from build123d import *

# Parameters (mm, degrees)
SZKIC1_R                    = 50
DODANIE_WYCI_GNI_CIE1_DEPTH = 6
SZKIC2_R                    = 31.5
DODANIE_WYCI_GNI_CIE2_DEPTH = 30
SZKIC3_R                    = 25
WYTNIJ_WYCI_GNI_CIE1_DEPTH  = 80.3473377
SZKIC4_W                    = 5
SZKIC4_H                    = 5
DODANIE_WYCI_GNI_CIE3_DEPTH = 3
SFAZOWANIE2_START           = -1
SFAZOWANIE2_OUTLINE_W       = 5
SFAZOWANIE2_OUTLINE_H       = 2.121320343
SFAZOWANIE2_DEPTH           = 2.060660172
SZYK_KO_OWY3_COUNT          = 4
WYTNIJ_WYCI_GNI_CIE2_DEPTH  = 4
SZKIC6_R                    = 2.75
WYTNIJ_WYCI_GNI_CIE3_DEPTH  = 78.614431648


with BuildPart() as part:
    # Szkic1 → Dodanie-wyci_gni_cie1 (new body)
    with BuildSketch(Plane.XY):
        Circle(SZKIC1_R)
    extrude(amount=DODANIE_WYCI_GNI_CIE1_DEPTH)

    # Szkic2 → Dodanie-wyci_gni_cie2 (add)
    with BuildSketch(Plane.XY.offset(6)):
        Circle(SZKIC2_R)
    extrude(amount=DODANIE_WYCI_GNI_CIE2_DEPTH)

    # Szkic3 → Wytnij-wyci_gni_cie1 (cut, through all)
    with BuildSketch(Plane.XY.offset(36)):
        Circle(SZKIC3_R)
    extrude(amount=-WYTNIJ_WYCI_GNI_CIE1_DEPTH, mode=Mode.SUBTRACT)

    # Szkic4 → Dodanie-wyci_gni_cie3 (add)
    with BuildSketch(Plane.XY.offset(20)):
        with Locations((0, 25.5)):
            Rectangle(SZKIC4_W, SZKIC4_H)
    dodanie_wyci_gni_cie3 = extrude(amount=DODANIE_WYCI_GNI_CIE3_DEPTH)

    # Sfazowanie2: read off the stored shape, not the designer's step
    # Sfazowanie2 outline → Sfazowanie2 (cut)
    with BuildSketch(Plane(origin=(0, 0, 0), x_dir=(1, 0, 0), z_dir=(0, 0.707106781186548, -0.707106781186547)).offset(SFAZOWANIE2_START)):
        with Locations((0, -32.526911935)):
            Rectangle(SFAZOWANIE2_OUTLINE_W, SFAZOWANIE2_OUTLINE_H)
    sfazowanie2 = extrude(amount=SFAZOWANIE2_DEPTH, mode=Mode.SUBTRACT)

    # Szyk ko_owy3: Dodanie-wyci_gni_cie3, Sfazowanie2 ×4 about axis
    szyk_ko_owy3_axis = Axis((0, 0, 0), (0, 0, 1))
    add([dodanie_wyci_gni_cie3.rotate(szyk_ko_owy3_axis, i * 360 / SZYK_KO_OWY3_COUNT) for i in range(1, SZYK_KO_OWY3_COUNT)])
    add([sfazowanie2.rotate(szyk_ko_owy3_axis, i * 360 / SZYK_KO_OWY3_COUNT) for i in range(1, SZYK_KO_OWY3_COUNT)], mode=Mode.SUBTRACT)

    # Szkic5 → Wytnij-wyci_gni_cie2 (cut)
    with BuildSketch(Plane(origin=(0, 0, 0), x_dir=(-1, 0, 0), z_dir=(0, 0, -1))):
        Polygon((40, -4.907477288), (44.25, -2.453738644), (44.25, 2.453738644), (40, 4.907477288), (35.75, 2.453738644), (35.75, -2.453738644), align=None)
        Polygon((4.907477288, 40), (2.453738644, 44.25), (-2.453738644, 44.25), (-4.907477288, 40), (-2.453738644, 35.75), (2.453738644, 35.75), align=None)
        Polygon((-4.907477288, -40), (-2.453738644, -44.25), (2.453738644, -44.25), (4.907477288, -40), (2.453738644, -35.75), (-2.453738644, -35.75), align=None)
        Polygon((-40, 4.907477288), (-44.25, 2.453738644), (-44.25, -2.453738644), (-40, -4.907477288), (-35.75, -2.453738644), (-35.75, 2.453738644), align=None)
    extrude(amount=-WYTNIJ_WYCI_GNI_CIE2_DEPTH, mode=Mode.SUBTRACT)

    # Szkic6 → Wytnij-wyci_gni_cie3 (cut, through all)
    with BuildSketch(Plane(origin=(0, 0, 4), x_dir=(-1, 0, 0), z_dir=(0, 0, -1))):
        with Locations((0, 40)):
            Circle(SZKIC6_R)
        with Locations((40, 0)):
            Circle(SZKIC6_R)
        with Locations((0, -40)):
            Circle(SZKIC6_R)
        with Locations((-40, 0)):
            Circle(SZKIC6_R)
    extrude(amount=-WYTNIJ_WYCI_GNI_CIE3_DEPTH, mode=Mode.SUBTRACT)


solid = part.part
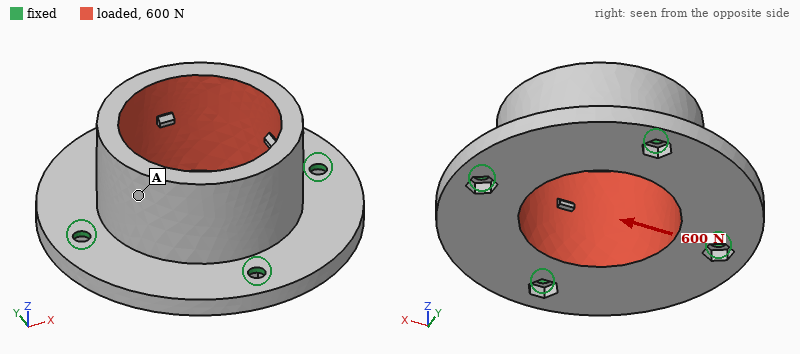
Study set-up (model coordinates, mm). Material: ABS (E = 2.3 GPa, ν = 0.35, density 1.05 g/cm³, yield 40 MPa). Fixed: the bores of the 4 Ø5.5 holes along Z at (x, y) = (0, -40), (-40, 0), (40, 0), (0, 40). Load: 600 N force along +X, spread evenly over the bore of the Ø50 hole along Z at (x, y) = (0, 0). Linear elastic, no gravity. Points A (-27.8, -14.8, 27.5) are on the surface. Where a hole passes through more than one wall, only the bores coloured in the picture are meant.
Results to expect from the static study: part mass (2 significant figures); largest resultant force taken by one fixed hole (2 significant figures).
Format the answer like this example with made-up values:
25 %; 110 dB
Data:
72 g; 180 N
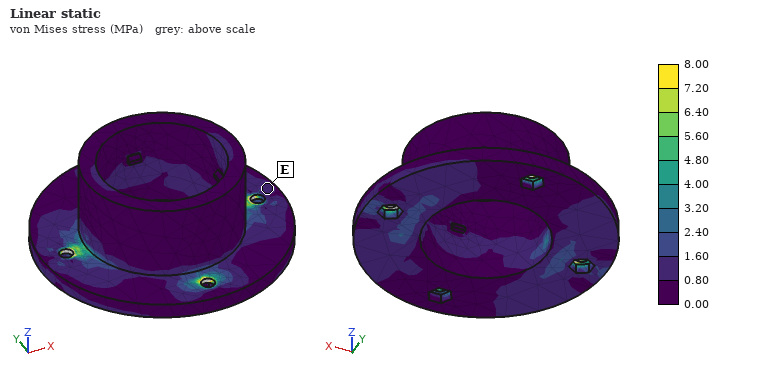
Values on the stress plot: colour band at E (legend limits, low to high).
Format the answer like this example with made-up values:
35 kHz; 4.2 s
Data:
0.80 to 1.60 MPa
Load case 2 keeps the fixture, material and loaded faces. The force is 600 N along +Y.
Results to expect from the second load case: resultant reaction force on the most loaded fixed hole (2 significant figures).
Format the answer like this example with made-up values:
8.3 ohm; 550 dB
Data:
180 N
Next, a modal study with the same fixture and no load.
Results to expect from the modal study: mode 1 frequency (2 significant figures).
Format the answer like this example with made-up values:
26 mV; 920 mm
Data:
1600 Hz
